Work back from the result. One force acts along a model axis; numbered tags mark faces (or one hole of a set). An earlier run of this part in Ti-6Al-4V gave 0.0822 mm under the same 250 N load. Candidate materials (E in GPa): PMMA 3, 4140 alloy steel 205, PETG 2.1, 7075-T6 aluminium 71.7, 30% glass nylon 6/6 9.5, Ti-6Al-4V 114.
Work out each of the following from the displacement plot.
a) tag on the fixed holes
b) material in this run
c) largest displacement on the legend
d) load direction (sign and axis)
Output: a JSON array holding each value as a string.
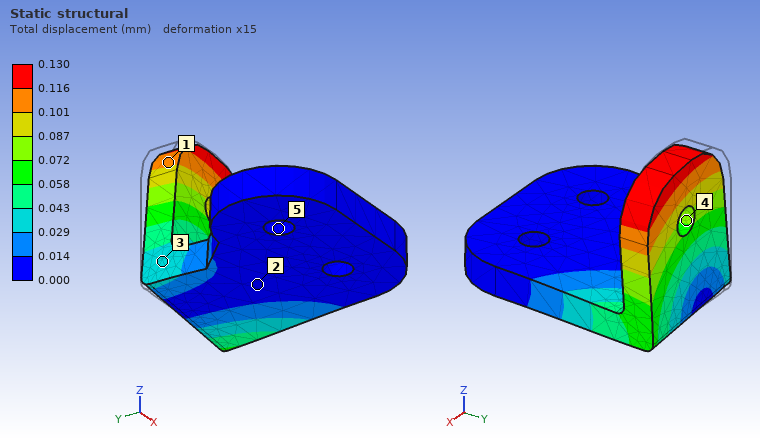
["5", "7075-T6 aluminium", "0.130 mm", "+X"]
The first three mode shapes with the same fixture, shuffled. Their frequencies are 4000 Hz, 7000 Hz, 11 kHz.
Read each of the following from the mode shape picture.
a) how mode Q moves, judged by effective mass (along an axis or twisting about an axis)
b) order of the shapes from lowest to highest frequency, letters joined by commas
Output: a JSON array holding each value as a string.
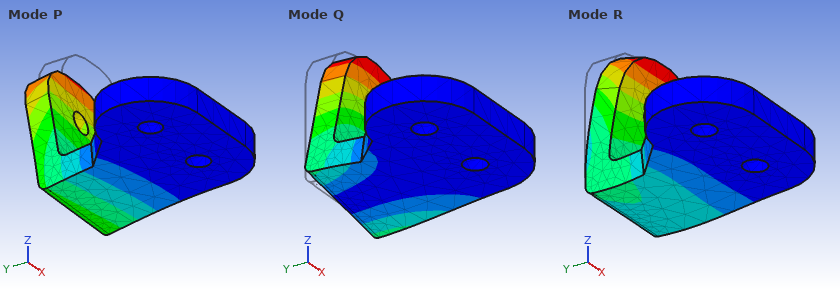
["along X", "P, Q, R"]
